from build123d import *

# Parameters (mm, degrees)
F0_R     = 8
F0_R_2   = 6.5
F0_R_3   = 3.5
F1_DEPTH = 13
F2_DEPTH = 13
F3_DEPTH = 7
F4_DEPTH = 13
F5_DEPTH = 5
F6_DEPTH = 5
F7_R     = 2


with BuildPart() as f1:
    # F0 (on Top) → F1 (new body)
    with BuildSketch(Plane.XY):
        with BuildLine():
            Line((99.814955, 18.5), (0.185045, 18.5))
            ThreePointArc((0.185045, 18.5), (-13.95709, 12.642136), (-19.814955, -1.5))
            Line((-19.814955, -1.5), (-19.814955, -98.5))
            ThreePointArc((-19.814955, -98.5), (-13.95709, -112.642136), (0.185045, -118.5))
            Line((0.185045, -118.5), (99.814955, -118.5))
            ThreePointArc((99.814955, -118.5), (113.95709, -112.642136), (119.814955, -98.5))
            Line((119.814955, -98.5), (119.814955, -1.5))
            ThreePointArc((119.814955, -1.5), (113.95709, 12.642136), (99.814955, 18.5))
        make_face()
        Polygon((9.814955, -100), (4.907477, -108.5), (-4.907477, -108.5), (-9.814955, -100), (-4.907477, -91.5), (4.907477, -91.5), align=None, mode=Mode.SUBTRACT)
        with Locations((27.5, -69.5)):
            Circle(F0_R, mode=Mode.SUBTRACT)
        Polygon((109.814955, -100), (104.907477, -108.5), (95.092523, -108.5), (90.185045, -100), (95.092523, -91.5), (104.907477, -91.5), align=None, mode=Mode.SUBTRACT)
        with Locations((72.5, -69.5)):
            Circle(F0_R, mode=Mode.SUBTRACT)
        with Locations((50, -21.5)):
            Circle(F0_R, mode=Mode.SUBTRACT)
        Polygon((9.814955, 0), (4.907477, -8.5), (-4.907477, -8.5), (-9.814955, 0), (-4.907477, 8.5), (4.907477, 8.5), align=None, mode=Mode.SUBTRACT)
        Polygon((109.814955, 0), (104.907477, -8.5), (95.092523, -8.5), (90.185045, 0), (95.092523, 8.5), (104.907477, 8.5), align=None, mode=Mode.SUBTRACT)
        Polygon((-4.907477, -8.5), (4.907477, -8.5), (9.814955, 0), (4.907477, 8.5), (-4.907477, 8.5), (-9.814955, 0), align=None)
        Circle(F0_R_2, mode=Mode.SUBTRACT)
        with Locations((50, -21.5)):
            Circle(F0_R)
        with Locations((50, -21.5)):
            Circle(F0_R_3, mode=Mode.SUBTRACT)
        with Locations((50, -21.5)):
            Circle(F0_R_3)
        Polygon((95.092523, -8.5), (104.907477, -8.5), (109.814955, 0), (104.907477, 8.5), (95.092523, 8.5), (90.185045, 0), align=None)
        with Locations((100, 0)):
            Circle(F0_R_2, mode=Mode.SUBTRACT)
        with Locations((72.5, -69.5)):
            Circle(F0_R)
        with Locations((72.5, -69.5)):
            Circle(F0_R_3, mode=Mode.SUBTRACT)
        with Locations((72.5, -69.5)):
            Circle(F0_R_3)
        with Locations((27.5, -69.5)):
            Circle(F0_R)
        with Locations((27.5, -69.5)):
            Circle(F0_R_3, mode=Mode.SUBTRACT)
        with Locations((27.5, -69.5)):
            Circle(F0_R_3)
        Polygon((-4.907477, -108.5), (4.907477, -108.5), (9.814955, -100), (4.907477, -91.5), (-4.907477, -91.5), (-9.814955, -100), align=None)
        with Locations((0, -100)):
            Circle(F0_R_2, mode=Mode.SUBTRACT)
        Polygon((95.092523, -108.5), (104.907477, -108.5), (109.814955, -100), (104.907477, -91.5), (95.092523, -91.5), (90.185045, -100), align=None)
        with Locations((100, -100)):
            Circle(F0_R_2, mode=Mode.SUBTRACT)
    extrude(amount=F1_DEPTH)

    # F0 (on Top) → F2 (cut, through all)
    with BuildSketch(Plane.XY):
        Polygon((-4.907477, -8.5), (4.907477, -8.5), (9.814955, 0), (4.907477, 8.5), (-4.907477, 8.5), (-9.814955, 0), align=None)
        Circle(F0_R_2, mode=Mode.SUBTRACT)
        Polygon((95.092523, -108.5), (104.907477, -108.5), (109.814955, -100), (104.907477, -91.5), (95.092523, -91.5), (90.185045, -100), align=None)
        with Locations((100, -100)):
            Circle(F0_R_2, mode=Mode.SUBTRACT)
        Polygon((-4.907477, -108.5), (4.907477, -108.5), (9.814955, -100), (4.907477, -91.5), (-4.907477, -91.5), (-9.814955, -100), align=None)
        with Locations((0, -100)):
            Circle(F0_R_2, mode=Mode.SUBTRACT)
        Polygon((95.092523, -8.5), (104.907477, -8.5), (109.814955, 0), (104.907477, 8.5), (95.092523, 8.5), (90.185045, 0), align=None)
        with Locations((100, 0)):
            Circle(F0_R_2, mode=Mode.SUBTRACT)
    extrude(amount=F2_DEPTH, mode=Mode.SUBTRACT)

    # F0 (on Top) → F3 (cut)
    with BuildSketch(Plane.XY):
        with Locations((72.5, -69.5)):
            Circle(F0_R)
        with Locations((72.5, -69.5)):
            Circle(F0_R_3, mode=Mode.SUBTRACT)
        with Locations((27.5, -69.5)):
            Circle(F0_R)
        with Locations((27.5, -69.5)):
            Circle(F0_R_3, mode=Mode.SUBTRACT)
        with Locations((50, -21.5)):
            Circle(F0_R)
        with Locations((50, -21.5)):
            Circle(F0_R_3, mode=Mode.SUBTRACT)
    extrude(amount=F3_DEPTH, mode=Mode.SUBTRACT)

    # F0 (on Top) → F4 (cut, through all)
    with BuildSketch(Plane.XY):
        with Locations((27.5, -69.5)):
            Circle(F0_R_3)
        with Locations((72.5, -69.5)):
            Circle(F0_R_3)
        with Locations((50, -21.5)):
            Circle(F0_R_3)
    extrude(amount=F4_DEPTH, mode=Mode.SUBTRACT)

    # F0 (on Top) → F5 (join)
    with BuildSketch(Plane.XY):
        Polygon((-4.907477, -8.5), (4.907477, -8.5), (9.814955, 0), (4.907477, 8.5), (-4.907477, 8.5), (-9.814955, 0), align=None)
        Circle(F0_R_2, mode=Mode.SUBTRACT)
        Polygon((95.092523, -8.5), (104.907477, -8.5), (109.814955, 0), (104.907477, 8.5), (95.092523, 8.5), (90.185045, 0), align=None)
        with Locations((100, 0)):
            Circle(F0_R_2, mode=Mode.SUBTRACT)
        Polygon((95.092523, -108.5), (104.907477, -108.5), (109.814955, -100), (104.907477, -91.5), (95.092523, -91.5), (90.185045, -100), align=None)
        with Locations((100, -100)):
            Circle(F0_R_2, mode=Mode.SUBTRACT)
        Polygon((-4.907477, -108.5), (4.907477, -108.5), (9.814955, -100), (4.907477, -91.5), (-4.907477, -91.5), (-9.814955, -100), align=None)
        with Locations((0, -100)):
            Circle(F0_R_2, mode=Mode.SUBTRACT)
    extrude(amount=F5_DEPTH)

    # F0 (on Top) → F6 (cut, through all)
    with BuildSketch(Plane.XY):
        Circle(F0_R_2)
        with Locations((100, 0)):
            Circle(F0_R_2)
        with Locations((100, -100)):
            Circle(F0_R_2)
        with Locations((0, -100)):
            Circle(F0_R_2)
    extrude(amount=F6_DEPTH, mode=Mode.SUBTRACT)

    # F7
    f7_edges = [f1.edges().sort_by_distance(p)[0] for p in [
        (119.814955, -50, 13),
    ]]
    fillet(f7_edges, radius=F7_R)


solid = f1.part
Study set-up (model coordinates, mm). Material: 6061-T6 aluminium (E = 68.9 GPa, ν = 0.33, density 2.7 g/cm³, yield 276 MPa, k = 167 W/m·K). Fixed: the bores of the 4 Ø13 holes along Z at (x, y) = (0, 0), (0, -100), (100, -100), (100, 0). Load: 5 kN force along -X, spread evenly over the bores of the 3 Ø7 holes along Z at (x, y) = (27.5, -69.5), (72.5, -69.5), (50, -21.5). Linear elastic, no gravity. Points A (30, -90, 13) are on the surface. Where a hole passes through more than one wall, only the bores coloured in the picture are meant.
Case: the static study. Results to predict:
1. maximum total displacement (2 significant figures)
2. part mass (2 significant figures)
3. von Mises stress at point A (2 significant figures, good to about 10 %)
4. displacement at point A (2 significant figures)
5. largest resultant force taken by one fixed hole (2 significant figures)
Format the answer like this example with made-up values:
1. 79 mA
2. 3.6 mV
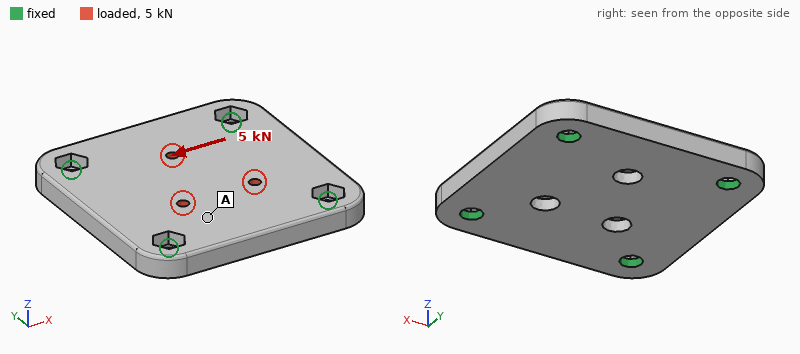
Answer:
1. 4.6 µm
2. 620 g
3. 2.5 MPa
4. 1.9 µm
5. 1.4 kN
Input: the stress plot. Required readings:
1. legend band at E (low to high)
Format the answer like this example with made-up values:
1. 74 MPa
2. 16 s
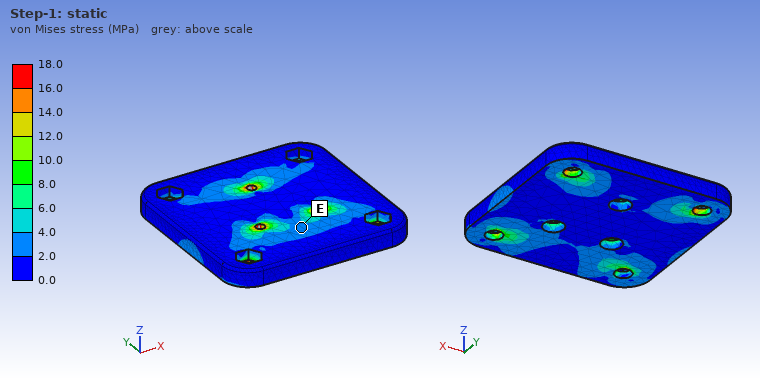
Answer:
1. 2.0 to 4.0 MPa
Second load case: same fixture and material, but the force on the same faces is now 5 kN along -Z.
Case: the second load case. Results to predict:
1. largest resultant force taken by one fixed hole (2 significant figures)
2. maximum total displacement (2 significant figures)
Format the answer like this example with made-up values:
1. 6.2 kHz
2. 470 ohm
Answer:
1. 2.4 kN
2. 43 µm
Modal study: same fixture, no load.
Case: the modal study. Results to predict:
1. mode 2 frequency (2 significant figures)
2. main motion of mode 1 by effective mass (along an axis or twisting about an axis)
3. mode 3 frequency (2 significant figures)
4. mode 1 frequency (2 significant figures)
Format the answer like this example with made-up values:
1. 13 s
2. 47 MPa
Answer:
1. 5500 Hz
2. along Z
3. 5600 Hz
4. 3900 Hz
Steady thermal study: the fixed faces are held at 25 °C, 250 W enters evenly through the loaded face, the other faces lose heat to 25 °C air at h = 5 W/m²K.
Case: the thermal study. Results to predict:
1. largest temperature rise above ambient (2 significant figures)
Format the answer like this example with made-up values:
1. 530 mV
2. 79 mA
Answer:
1. 44 K
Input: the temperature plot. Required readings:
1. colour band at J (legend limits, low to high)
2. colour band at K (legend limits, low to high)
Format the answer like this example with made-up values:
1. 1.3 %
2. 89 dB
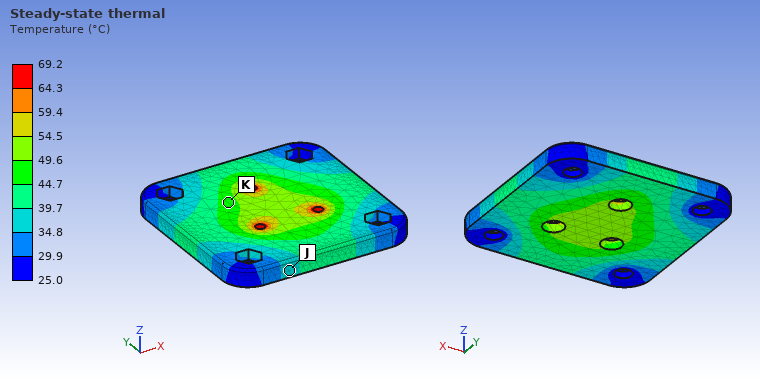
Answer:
1. 34.8 to 39.7 °C
2. 44.7 to 49.6 °C
